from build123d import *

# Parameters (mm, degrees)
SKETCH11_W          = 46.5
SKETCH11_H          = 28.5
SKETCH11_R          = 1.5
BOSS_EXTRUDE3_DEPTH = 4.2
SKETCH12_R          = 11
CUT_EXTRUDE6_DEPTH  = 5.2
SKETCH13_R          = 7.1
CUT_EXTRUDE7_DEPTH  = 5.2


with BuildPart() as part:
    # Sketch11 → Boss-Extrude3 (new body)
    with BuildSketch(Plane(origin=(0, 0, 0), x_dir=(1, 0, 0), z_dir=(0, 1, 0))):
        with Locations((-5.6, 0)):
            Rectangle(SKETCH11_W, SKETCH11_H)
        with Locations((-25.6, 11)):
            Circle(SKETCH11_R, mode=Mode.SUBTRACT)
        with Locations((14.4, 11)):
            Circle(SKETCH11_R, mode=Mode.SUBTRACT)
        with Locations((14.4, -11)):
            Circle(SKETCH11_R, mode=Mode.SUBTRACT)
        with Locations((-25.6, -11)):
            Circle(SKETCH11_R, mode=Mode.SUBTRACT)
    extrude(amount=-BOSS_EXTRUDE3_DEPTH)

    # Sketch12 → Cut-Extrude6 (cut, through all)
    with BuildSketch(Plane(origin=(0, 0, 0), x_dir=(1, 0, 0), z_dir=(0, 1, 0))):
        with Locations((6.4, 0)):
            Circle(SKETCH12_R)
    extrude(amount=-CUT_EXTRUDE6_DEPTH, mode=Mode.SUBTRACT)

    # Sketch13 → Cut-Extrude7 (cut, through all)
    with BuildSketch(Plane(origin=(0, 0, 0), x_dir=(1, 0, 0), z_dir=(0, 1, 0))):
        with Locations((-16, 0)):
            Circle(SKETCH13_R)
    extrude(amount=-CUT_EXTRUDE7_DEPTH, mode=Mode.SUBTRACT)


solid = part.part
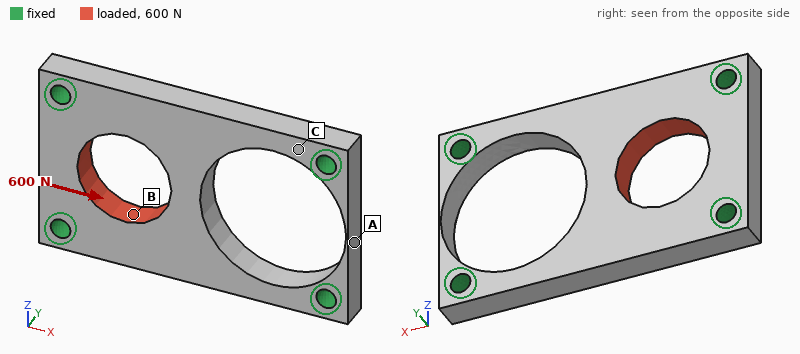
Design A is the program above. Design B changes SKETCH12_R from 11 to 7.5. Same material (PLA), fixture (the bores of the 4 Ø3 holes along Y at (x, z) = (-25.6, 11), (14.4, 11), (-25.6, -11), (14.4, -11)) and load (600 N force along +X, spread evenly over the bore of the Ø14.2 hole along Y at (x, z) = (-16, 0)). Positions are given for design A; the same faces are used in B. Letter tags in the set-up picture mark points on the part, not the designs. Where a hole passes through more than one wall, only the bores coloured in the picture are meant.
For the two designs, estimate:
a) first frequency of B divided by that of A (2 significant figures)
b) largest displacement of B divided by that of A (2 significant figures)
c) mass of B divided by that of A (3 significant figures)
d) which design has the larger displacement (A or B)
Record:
1.1
0.69
1.27
A
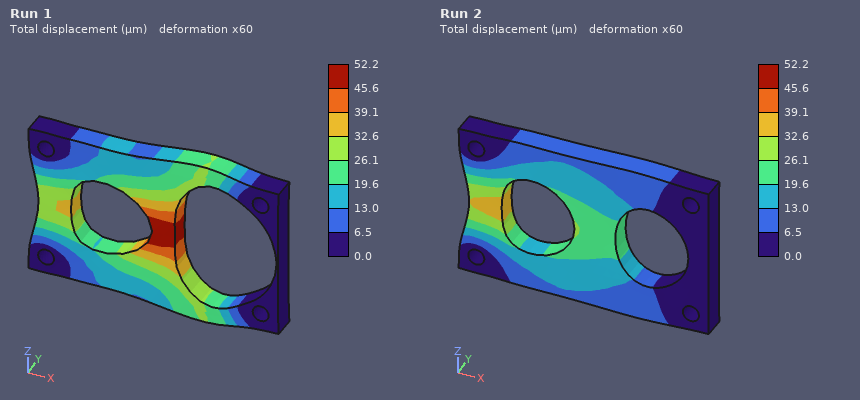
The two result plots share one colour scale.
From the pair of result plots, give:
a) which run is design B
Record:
Run 2
